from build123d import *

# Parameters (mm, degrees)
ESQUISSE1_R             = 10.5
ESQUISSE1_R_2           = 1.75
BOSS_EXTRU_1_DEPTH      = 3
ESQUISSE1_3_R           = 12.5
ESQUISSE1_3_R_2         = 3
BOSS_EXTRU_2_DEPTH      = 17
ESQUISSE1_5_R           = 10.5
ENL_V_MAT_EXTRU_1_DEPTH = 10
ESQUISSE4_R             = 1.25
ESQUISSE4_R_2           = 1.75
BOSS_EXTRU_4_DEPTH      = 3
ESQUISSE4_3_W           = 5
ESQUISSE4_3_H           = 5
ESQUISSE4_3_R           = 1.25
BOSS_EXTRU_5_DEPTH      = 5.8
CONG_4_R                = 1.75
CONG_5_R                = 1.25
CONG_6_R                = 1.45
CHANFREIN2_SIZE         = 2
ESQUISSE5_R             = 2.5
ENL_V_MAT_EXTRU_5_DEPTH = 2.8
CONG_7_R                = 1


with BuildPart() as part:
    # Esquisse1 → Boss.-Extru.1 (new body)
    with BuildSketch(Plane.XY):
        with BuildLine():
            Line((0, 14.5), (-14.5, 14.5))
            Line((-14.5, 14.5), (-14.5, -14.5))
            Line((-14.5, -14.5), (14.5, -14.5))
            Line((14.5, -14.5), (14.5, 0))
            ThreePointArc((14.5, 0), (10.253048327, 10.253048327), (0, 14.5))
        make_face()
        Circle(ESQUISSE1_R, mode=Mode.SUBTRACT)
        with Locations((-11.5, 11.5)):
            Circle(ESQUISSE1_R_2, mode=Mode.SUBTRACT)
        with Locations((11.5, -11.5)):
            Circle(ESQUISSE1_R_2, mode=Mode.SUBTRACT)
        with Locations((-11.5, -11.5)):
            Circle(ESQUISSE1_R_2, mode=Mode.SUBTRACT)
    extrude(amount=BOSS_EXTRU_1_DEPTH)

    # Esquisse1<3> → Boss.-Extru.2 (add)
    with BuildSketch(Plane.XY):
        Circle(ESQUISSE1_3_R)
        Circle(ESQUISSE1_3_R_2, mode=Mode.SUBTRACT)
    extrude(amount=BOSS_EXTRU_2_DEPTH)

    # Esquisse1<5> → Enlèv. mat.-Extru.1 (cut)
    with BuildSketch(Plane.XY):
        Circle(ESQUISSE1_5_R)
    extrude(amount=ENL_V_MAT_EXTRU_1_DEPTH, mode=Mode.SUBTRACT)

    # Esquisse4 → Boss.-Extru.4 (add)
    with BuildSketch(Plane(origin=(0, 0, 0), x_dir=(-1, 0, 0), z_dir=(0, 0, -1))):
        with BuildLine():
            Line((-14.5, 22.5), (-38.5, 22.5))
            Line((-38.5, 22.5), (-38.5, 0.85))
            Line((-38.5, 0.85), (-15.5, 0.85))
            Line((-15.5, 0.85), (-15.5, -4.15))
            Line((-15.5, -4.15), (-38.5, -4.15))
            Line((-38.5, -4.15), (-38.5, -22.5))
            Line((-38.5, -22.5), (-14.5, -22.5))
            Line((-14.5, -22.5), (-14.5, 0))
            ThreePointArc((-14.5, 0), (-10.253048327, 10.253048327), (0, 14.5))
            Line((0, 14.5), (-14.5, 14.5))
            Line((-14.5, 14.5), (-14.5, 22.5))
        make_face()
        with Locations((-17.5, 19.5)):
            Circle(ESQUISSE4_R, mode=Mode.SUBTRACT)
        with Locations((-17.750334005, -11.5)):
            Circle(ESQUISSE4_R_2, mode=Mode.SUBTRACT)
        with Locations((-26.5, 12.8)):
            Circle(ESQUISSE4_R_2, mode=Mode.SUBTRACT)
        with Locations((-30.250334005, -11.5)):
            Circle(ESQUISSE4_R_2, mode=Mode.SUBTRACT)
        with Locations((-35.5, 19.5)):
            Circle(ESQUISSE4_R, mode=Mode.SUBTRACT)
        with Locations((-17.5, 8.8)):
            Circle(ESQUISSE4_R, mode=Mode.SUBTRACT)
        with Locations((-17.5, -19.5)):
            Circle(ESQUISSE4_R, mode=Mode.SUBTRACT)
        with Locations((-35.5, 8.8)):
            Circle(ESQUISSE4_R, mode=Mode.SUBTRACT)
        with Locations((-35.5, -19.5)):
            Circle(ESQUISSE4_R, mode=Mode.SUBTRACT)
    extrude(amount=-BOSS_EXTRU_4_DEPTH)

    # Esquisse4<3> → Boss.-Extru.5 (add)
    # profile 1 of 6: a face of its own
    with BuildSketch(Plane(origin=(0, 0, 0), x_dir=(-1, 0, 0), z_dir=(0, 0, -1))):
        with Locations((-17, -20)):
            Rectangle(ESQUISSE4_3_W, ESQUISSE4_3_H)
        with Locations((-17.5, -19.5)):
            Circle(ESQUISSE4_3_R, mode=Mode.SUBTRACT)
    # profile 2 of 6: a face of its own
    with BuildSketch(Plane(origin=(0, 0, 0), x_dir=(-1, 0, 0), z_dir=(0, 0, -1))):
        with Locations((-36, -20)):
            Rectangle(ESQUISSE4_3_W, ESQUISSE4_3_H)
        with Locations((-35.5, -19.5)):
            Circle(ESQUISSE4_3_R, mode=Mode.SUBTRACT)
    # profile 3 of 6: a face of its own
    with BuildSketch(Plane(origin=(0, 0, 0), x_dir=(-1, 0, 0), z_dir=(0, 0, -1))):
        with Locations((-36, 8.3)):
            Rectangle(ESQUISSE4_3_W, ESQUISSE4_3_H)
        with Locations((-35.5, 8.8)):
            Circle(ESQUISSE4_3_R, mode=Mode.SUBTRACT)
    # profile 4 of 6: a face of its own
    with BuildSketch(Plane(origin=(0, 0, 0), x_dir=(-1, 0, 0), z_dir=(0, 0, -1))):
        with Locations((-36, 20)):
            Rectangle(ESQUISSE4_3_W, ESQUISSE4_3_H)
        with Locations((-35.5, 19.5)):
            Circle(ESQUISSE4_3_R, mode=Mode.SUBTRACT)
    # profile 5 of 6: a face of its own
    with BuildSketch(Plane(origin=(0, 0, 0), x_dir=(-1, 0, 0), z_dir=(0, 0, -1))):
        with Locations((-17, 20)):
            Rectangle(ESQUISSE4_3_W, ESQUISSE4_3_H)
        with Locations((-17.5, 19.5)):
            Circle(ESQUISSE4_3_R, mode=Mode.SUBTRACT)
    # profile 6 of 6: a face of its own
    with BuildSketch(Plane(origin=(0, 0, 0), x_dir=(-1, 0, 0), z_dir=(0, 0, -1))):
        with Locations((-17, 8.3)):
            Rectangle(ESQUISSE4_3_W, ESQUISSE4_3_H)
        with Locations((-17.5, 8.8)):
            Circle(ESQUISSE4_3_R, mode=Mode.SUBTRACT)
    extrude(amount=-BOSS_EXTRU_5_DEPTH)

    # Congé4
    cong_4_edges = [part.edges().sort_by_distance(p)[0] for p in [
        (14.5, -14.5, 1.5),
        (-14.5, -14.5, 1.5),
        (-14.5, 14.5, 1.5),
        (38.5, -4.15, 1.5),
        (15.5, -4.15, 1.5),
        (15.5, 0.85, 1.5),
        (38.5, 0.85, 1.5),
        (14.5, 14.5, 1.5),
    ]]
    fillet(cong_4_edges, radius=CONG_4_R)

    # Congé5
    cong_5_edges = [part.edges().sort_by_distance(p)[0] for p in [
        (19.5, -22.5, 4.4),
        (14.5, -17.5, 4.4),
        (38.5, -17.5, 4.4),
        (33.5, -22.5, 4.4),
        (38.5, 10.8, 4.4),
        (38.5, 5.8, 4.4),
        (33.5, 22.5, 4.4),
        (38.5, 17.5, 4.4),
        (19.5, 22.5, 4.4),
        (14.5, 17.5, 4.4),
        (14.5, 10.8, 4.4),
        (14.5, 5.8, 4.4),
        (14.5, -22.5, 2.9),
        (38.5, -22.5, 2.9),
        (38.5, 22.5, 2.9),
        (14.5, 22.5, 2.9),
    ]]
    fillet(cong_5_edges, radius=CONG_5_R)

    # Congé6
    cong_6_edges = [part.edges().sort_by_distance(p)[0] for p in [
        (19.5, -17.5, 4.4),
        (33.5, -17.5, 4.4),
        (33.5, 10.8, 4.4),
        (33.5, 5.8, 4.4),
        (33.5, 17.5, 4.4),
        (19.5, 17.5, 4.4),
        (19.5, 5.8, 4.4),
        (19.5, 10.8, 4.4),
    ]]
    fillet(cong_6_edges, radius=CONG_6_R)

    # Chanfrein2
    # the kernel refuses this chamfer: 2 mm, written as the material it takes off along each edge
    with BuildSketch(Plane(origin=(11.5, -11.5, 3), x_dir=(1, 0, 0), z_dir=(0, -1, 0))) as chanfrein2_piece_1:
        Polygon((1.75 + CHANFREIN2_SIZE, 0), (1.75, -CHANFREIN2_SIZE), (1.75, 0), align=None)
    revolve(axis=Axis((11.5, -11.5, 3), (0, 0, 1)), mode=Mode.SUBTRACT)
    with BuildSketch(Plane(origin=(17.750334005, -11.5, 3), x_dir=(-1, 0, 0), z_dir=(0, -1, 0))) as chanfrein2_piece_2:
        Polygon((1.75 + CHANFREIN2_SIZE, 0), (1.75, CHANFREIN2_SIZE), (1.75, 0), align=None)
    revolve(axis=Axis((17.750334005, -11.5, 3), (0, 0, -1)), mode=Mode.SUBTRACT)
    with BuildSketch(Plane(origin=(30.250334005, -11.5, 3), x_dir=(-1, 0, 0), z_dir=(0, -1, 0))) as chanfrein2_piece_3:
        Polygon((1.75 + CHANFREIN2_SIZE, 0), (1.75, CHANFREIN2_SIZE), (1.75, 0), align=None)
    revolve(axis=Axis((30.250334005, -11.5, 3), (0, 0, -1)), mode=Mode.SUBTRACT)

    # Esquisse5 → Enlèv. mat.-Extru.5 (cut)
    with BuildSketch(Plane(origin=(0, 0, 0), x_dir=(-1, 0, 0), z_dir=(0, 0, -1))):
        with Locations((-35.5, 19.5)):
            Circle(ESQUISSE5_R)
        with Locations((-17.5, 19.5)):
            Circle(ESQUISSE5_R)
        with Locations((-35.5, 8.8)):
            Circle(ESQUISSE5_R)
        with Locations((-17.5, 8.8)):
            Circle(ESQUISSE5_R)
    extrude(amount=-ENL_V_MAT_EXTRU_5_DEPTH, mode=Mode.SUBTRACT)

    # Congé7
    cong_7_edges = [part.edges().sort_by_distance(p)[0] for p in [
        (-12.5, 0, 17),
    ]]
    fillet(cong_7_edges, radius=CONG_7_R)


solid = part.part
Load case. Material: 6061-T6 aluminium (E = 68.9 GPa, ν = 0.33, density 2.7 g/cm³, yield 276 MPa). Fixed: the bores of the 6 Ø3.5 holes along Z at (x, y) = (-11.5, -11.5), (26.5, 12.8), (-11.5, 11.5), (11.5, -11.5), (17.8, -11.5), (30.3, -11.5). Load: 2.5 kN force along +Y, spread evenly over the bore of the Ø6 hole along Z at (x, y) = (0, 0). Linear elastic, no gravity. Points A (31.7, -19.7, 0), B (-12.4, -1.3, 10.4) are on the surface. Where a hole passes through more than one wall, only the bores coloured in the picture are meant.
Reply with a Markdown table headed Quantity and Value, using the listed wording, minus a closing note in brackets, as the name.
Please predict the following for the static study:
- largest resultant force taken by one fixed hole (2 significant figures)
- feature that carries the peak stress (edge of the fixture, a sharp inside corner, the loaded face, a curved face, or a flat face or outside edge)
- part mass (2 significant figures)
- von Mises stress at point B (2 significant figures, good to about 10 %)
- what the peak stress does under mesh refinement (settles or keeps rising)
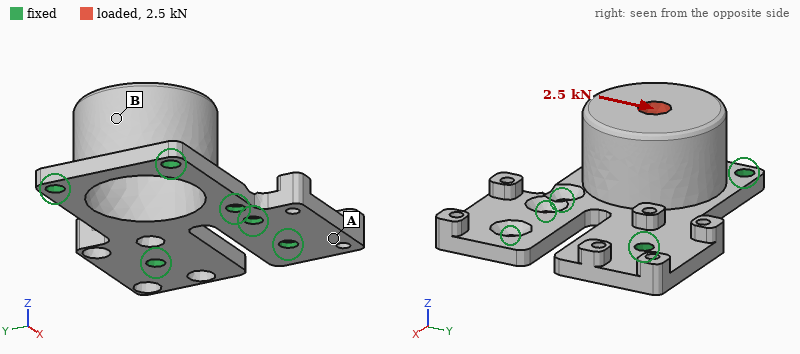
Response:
| Quantity | Value |
|---|---|
| largest resultant force taken by one fixed hole | 1.5 kN |
| feature that carries the peak stress | edge of the fixture |
| part mass | 23 g |
| von Mises stress at point B | 46 MPa |
| what the peak stress does under mesh refinement | keeps rising |
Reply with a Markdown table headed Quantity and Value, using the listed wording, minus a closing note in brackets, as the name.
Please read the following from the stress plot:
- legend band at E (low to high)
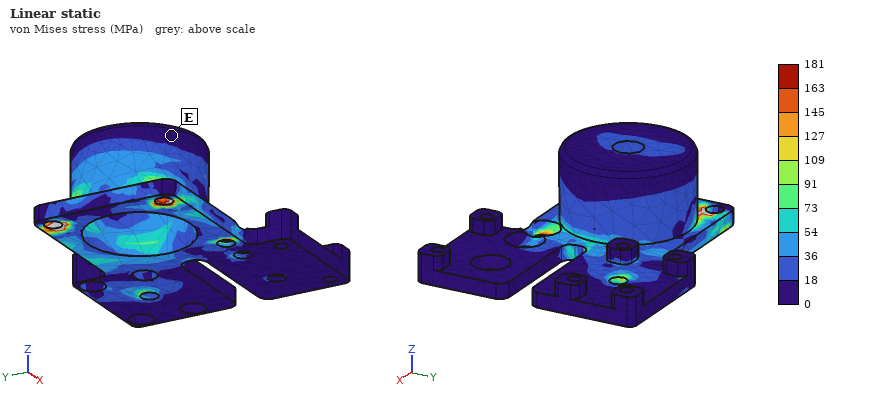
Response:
| Quantity | Value |
|---|---|
| legend band at E | 0 to 18 MPa |
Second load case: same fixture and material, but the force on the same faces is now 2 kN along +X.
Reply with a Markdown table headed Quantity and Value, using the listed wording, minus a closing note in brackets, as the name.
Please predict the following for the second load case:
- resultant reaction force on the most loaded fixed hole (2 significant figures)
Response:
| Quantity | Value |
|---|---|
| resultant reaction force on the most loaded fixed hole | 1.0 kN |
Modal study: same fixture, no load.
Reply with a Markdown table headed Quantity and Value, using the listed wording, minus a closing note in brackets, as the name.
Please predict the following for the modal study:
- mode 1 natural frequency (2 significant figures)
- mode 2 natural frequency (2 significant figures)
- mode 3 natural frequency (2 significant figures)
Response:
| Quantity | Value |
|---|---|
| mode 1 natural frequency | 9100 Hz |
| mode 2 natural frequency | 11 kHz |
| mode 3 natural frequency | 13 kHz |
